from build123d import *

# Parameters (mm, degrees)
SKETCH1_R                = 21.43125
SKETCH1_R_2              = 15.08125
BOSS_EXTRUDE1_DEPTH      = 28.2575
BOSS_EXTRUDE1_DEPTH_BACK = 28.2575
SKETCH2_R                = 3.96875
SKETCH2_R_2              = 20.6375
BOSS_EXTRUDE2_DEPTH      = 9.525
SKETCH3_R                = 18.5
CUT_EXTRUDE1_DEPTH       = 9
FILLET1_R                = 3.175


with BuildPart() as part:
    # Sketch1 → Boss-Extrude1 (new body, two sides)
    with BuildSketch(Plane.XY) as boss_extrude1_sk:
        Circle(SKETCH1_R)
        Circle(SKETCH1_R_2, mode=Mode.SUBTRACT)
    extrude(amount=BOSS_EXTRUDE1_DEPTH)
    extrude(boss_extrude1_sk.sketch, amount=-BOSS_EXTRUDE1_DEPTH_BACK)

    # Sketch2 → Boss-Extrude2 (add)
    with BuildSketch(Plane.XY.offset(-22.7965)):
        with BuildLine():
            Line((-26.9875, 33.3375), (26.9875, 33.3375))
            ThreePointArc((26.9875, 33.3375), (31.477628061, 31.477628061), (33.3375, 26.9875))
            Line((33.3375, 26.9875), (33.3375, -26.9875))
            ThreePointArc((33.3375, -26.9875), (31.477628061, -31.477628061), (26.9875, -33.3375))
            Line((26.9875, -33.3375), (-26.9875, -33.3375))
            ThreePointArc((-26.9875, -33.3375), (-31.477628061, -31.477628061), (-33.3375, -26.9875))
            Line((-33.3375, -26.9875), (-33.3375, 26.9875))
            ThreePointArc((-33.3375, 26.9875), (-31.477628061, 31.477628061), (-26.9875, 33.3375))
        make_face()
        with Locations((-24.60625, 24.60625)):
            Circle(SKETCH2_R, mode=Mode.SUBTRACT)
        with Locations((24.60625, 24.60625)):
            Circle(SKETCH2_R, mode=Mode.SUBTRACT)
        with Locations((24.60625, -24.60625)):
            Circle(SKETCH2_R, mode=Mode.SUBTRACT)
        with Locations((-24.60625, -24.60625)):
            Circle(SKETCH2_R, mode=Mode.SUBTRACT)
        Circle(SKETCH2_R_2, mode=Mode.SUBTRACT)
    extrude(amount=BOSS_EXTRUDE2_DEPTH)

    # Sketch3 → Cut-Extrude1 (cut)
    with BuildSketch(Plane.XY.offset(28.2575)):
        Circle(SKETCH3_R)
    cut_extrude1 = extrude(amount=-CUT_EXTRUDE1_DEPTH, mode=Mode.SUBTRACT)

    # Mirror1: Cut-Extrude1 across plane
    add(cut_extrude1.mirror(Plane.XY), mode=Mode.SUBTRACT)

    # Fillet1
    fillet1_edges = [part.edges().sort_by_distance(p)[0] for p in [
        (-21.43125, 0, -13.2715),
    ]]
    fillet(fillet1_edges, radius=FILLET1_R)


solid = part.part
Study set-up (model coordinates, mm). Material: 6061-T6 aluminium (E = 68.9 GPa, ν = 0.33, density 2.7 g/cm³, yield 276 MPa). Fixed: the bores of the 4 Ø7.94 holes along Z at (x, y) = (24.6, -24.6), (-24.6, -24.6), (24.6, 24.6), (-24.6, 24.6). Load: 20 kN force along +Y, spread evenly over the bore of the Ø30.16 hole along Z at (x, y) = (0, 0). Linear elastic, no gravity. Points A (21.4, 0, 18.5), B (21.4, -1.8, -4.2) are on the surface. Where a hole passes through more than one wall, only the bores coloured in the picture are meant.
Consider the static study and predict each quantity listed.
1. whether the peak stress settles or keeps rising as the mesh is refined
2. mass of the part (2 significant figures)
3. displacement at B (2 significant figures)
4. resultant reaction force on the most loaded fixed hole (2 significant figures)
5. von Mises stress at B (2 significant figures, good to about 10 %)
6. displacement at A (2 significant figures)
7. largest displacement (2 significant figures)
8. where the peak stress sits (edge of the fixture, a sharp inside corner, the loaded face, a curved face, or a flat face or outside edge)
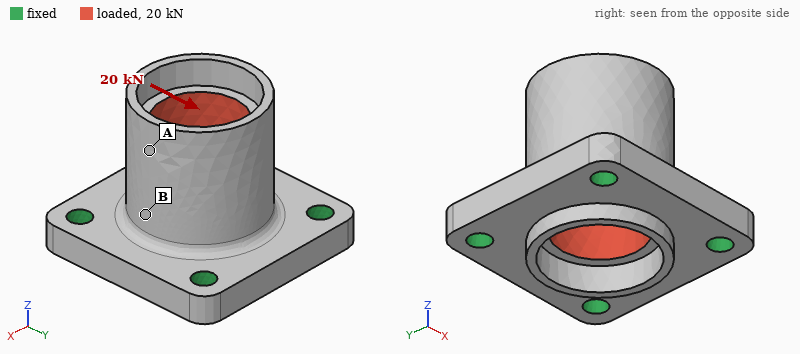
keeps rising
170 g
31 µm
6.7 kN
36 MPa
74 µm
92 µm
edge of the fixture
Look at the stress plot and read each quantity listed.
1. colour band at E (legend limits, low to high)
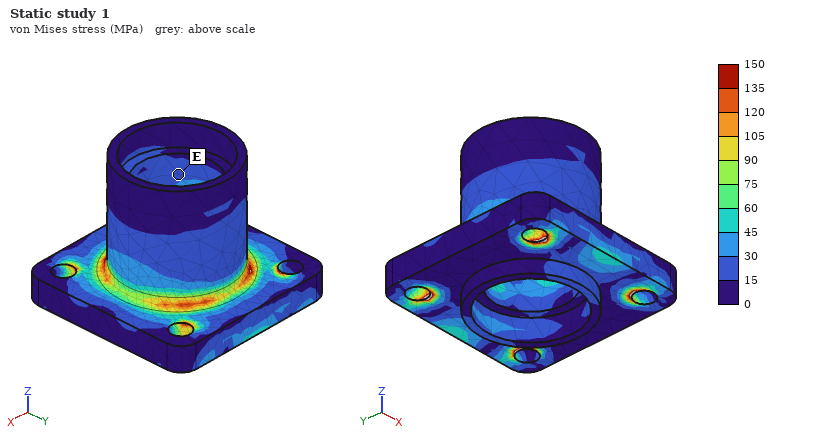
15 to 30 MPa
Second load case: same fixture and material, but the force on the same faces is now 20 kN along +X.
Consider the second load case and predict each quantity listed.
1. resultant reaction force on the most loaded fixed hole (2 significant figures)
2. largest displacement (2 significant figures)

6.7 kN
92 µm
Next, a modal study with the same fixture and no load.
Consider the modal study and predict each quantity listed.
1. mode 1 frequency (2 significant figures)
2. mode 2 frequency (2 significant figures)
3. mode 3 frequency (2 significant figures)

8300 Hz
8300 Hz
12 kHz
